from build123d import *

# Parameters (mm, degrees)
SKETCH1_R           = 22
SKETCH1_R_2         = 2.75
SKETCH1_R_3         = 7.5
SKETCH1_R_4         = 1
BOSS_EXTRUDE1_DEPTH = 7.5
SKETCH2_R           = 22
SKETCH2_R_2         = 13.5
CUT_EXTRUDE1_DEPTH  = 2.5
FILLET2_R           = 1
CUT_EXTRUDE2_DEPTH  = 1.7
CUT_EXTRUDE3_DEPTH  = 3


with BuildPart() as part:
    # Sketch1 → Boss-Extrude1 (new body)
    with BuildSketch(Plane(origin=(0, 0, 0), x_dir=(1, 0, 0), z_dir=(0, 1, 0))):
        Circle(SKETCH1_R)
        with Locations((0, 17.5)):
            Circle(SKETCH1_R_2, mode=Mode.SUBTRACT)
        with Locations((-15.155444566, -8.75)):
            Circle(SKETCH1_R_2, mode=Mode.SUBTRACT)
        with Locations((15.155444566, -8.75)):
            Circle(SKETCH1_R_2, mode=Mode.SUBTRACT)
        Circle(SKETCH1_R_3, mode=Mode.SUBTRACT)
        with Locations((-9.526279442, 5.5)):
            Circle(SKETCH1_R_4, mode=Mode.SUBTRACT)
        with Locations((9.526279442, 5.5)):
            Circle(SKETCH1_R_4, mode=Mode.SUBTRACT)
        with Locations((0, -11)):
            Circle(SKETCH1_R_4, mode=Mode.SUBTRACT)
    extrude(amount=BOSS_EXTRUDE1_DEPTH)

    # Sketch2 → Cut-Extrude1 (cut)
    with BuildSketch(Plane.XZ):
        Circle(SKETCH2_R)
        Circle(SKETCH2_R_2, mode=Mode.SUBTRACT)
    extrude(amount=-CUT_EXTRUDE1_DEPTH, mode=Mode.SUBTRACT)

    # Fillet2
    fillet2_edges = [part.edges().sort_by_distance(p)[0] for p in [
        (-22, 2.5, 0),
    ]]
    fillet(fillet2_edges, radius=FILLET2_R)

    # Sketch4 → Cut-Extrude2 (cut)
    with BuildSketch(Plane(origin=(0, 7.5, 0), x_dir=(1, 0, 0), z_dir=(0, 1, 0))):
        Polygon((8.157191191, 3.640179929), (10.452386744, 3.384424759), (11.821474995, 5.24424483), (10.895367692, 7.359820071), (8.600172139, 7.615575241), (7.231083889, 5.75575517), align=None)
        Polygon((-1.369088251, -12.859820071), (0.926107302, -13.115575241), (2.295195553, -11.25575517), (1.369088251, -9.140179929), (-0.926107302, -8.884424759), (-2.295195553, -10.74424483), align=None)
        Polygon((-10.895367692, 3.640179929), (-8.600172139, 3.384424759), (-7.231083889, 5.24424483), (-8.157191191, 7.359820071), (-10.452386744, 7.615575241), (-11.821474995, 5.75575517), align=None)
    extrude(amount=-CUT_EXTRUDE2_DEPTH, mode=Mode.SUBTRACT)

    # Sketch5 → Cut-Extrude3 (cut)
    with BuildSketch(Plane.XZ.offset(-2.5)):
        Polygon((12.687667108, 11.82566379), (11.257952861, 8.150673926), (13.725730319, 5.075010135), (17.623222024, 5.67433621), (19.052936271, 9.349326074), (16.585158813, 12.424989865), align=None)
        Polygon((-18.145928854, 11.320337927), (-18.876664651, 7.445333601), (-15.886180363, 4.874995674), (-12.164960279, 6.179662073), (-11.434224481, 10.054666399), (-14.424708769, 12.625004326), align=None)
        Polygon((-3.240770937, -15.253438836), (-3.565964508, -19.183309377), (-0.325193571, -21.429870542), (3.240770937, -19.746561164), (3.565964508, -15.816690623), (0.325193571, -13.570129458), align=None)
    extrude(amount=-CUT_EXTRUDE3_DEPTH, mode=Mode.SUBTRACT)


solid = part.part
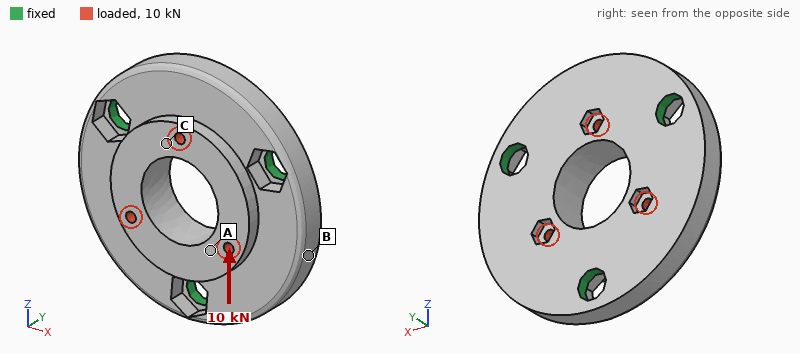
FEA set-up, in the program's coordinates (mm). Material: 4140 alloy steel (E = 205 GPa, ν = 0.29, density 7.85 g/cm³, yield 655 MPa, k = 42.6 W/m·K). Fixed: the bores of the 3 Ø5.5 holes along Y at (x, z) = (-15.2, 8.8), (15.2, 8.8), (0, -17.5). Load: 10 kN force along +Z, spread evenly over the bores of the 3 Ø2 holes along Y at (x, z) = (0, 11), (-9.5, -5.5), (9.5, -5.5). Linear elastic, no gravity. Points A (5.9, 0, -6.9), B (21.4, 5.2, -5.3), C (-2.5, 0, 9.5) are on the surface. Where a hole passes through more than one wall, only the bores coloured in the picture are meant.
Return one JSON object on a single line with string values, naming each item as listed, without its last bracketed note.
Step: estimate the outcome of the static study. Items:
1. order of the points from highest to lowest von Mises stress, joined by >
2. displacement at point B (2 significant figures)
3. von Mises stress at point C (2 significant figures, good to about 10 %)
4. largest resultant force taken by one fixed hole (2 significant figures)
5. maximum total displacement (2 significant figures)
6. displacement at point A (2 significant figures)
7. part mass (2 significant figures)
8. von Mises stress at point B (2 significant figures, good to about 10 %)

{"order of the points from highest to lowest von Mises stress, joined by >": "C > A > B", "displacement at point B": "8.4 µm", "von Mises stress at point C": "98 MPa", "largest resultant force taken by one fixed hole": "3.5 kN", "maximum total displacement": "18 µm", "displacement at point A": "5.6 µm", "part mass": "55 g", "von Mises stress at point B": "24 MPa"}
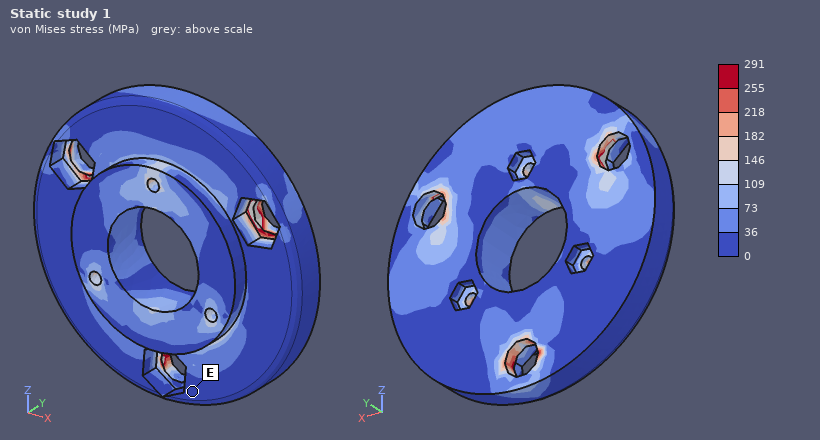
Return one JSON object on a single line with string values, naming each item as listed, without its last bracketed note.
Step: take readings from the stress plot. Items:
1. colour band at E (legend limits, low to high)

{"colour band at E": "0 to 36 MPa"}
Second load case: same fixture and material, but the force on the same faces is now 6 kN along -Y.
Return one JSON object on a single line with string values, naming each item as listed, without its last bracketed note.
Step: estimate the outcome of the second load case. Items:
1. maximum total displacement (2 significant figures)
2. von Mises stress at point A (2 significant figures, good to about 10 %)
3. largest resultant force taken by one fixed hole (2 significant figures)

{"maximum total displacement": "12 µm", "von Mises stress at point A": "90 MPa", "largest resultant force taken by one fixed hole": "2.7 kN"}
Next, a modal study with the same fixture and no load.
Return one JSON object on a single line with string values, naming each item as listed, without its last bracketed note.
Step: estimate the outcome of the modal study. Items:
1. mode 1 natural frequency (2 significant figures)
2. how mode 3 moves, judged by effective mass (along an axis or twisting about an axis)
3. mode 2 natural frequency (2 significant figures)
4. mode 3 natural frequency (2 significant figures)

{"mode 1 natural frequency": "16 kHz", "how mode 3 moves, judged by effective mass": "along Y", "mode 2 natural frequency": "16 kHz", "mode 3 natural frequency": "20 kHz"}
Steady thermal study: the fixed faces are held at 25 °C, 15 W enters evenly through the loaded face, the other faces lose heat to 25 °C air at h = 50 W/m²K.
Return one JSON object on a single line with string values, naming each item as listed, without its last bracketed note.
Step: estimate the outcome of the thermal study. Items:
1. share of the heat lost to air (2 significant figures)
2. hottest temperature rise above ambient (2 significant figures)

{"share of the heat lost to air": "12 %", "hottest temperature rise above ambient": "19 K"}
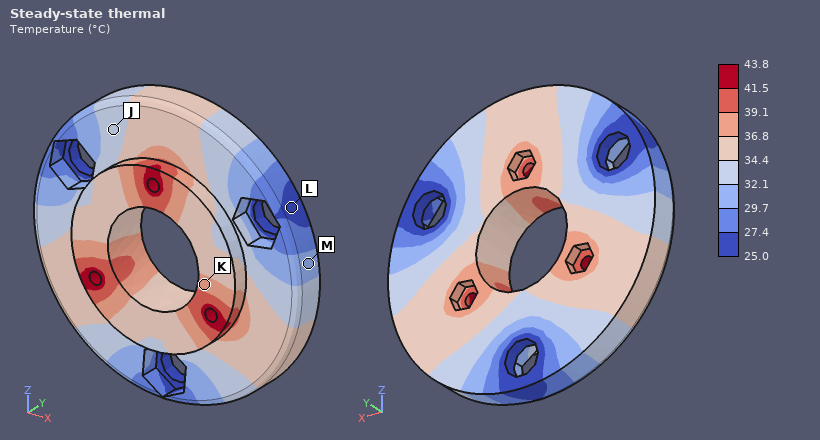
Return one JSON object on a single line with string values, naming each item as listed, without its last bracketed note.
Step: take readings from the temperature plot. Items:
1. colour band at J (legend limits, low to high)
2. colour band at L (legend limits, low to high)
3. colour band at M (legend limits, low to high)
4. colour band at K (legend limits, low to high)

{"colour band at J": "32.1 to 34.4 °C", "colour band at L": "25.0 to 27.4 °C", "colour band at M": "29.7 to 32.1 °C", "colour band at K": "36.8 to 39.1 °C"}
